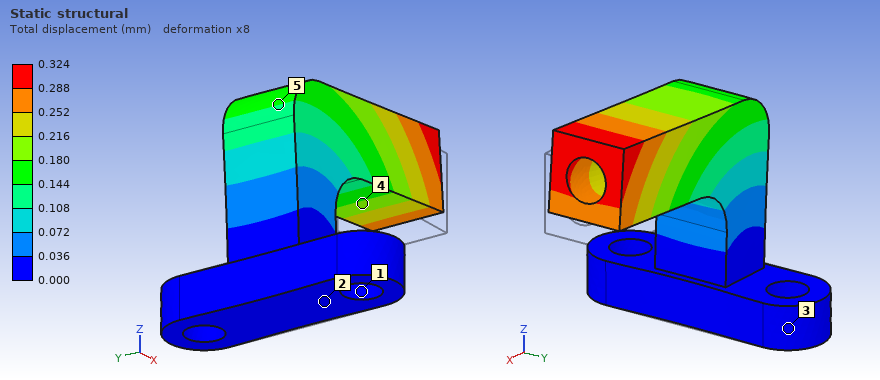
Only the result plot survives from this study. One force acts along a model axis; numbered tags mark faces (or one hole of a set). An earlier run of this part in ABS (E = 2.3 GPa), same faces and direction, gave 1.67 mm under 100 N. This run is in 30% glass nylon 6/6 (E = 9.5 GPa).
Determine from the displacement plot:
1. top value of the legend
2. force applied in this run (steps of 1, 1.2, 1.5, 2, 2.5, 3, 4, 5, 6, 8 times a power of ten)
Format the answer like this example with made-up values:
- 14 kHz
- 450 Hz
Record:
- 0.324 mm
- 80 N
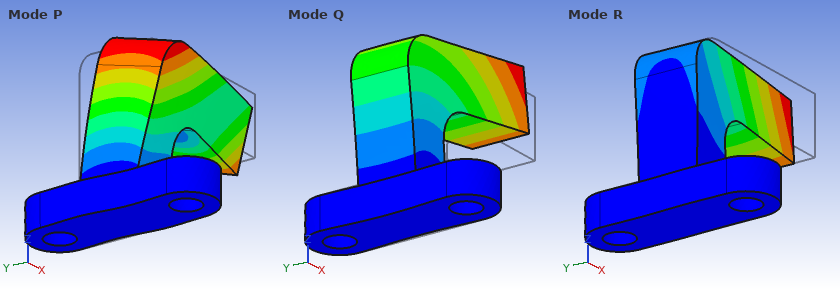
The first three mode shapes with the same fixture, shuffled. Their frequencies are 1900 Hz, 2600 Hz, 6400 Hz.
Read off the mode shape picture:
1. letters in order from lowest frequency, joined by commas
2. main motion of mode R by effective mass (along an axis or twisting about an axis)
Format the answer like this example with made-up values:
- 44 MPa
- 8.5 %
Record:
- Q, R, P
- along Y
